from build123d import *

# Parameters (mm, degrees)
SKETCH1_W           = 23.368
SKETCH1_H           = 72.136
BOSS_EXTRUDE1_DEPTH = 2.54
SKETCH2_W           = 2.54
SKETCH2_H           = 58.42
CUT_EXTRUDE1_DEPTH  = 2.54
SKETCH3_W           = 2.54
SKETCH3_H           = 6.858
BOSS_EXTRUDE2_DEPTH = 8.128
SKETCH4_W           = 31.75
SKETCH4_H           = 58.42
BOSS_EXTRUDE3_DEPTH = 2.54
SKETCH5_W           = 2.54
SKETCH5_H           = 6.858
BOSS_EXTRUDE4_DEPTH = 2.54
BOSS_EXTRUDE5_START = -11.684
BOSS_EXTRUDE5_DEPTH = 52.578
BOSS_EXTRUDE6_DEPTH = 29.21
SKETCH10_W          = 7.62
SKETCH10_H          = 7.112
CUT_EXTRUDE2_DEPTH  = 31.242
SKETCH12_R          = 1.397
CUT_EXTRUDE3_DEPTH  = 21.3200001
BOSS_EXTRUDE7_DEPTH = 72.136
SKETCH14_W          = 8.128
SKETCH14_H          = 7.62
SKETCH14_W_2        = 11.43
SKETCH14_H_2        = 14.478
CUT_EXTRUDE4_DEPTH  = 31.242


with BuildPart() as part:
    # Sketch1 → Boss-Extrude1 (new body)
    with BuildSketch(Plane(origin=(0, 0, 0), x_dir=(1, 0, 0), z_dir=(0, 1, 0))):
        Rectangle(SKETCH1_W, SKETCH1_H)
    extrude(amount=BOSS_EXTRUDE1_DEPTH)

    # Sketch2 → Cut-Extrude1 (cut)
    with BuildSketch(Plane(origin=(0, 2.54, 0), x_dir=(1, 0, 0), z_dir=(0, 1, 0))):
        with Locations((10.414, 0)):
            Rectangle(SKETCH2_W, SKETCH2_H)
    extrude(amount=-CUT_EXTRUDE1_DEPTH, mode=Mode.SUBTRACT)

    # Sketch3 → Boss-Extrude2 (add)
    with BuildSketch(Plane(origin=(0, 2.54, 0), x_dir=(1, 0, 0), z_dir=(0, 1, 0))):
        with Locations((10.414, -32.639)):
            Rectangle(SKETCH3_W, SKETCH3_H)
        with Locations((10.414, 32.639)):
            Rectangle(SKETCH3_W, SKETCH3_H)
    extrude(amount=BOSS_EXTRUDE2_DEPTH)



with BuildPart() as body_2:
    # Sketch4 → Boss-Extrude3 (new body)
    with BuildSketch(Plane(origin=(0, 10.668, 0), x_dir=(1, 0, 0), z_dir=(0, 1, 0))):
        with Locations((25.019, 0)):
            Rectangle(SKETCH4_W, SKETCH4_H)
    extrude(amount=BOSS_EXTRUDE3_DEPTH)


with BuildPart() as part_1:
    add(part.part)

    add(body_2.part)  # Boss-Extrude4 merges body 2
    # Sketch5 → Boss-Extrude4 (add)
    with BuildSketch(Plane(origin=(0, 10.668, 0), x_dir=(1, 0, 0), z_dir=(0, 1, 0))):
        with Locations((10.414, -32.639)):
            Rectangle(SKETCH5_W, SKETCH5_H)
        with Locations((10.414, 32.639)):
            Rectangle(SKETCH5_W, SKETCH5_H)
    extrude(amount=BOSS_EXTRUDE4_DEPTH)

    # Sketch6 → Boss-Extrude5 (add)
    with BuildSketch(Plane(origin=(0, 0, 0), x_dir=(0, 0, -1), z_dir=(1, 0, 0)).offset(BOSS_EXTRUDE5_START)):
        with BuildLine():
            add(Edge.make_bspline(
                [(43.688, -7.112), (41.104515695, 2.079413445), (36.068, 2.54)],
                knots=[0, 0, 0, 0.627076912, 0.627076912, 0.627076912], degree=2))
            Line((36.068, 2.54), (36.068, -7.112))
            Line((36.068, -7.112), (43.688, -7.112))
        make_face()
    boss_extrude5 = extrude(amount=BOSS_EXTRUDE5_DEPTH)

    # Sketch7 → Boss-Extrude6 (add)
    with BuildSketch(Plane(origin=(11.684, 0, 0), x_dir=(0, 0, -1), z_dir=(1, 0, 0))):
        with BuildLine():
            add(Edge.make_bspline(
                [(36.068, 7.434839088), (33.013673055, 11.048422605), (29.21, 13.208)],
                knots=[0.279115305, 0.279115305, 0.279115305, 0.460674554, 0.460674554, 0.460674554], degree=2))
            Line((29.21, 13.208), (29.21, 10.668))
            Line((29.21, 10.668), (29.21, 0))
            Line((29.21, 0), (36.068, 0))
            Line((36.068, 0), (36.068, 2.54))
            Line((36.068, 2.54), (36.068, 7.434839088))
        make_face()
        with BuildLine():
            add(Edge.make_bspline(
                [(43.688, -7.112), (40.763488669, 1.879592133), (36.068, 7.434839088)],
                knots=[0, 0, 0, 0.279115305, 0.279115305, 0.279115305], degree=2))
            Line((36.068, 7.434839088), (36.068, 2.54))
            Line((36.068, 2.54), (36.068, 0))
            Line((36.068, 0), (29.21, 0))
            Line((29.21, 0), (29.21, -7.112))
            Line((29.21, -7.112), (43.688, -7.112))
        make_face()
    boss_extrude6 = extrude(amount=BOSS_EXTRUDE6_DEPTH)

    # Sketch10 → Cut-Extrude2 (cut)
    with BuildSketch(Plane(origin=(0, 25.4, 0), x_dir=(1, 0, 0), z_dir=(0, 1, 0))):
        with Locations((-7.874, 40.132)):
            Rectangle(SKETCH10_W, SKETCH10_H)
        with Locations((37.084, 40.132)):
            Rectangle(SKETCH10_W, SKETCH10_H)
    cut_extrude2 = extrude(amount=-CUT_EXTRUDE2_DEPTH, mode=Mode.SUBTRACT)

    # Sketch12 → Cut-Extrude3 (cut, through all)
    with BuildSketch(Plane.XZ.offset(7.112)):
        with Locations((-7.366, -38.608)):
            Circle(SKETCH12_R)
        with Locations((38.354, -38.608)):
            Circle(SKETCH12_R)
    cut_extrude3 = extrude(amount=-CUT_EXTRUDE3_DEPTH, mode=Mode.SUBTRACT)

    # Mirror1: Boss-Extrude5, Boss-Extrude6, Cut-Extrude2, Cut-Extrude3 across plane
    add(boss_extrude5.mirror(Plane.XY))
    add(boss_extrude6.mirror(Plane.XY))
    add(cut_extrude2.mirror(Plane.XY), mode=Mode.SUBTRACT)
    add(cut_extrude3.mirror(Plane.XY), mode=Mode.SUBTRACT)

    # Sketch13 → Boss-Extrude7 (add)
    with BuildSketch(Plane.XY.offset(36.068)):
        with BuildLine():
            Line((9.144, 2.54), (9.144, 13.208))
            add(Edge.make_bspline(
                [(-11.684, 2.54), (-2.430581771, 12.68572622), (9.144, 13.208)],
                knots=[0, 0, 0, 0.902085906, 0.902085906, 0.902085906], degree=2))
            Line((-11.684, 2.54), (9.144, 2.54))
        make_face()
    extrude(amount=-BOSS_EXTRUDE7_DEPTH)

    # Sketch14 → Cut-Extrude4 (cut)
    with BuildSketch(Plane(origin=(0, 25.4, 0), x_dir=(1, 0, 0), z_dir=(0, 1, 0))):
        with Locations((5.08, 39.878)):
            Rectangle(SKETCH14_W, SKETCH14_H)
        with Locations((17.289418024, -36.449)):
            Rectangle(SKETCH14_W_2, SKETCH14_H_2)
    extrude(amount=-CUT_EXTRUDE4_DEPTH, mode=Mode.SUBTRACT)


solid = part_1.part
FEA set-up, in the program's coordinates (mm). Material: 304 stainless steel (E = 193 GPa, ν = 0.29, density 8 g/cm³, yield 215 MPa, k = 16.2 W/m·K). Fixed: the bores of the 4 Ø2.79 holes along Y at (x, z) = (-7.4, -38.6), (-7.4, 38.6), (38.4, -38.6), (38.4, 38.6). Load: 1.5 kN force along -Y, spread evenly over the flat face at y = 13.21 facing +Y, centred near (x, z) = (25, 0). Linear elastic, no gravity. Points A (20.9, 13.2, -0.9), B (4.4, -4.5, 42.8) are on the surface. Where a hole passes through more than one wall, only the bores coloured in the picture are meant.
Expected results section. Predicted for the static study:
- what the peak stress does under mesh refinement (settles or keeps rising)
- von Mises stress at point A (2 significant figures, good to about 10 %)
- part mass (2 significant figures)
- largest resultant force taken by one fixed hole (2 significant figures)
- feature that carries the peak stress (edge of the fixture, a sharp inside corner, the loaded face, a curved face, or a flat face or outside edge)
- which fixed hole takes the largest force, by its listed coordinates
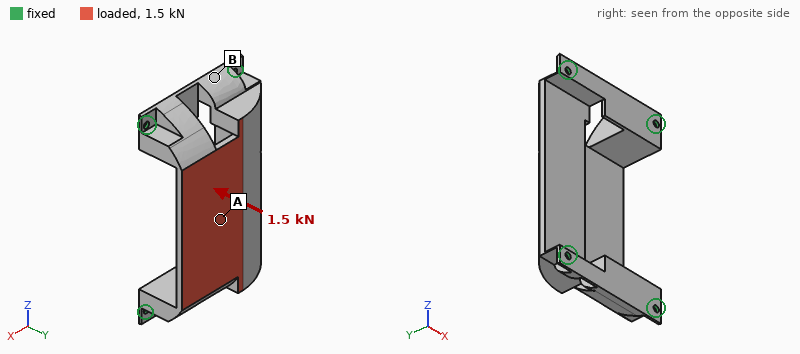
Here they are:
keeps rising
38 MPa
240 g
740 N
edge of the fixture
(38.4, -38.6)
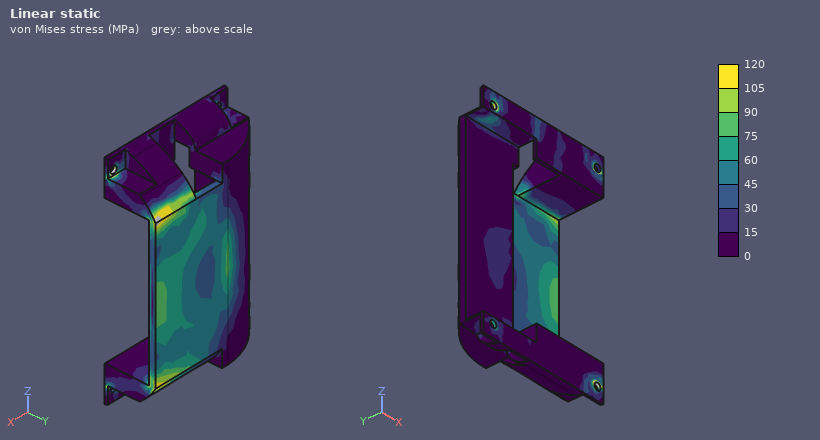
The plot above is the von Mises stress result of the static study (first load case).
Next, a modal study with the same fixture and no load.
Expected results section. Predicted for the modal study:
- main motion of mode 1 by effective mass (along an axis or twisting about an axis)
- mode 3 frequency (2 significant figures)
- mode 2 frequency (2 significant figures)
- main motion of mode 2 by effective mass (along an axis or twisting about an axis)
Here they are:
along Z
4700 Hz
3900 Hz
along Y
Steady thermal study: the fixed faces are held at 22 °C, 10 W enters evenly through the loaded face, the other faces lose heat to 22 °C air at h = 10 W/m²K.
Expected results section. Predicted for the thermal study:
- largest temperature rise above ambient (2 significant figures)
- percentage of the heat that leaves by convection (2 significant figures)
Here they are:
77 K
46 %
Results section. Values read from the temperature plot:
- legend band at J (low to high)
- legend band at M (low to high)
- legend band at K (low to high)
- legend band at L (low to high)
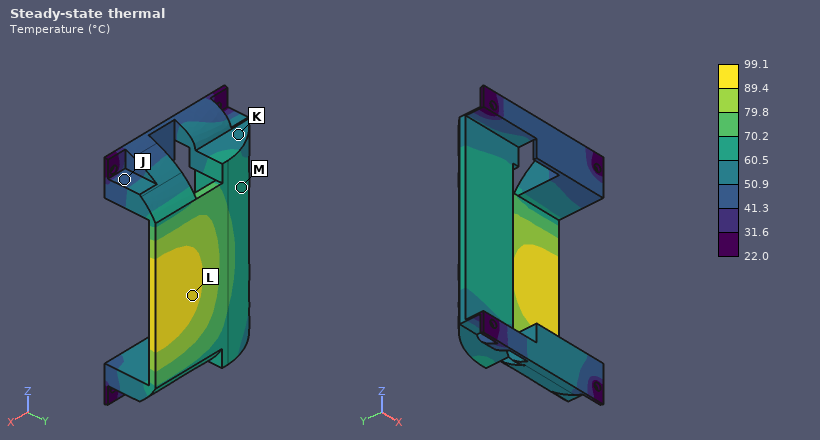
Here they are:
41.3 to 50.9 °C
60.5 to 70.2 °C
50.9 to 60.5 °C
89.4 to 99.1 °C
